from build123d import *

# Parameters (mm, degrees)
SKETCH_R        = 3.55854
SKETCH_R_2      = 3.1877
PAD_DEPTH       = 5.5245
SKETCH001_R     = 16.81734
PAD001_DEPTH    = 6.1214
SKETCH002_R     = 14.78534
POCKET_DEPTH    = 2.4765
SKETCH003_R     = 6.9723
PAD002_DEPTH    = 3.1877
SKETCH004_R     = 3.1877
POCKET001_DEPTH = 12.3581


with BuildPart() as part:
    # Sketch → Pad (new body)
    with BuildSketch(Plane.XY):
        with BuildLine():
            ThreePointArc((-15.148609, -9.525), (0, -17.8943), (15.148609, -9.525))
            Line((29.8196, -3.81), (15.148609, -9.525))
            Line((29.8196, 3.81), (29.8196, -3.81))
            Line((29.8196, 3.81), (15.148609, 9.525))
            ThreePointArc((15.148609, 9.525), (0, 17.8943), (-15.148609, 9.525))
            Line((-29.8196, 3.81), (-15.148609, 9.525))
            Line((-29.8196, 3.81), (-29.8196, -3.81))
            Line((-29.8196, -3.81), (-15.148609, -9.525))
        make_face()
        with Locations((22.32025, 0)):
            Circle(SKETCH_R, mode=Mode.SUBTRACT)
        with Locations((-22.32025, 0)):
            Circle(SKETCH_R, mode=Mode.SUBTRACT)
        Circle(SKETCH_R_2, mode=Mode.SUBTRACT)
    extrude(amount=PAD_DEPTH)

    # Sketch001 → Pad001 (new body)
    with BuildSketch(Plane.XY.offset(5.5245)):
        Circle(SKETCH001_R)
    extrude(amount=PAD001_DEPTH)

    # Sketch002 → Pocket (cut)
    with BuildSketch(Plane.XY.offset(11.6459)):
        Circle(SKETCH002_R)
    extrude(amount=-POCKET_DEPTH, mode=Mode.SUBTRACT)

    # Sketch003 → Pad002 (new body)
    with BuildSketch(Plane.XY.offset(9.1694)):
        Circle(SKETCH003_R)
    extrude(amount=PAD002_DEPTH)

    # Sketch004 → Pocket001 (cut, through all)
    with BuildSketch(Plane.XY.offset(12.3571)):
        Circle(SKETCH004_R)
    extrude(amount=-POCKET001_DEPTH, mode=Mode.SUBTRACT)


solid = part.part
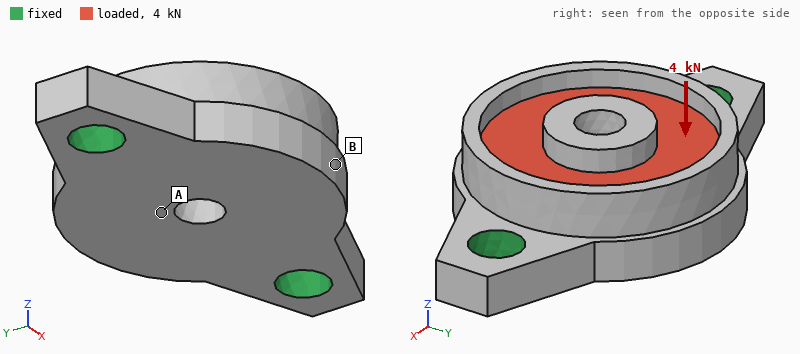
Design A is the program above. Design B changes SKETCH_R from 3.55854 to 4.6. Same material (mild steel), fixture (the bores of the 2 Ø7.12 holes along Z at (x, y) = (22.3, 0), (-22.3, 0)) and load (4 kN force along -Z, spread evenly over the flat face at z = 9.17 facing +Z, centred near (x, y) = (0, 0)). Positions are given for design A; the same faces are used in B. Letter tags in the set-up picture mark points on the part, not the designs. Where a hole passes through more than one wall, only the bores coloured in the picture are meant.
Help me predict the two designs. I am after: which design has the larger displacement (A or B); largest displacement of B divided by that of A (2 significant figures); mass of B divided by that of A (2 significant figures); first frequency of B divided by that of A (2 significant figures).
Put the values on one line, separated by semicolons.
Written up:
A; 0.84; 0.97; 1.2
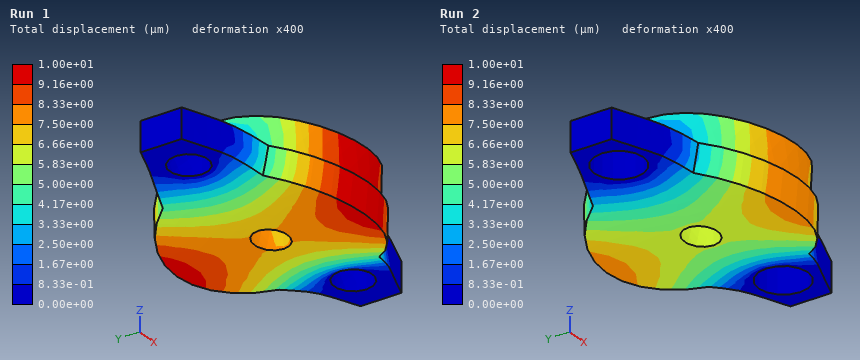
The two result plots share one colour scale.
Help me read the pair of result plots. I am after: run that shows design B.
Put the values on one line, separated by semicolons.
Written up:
Run 2
